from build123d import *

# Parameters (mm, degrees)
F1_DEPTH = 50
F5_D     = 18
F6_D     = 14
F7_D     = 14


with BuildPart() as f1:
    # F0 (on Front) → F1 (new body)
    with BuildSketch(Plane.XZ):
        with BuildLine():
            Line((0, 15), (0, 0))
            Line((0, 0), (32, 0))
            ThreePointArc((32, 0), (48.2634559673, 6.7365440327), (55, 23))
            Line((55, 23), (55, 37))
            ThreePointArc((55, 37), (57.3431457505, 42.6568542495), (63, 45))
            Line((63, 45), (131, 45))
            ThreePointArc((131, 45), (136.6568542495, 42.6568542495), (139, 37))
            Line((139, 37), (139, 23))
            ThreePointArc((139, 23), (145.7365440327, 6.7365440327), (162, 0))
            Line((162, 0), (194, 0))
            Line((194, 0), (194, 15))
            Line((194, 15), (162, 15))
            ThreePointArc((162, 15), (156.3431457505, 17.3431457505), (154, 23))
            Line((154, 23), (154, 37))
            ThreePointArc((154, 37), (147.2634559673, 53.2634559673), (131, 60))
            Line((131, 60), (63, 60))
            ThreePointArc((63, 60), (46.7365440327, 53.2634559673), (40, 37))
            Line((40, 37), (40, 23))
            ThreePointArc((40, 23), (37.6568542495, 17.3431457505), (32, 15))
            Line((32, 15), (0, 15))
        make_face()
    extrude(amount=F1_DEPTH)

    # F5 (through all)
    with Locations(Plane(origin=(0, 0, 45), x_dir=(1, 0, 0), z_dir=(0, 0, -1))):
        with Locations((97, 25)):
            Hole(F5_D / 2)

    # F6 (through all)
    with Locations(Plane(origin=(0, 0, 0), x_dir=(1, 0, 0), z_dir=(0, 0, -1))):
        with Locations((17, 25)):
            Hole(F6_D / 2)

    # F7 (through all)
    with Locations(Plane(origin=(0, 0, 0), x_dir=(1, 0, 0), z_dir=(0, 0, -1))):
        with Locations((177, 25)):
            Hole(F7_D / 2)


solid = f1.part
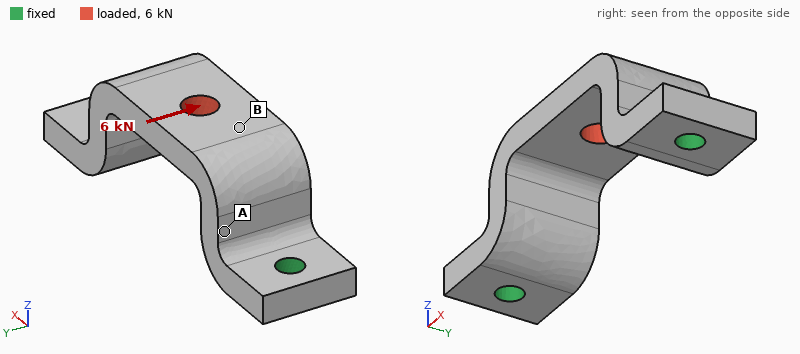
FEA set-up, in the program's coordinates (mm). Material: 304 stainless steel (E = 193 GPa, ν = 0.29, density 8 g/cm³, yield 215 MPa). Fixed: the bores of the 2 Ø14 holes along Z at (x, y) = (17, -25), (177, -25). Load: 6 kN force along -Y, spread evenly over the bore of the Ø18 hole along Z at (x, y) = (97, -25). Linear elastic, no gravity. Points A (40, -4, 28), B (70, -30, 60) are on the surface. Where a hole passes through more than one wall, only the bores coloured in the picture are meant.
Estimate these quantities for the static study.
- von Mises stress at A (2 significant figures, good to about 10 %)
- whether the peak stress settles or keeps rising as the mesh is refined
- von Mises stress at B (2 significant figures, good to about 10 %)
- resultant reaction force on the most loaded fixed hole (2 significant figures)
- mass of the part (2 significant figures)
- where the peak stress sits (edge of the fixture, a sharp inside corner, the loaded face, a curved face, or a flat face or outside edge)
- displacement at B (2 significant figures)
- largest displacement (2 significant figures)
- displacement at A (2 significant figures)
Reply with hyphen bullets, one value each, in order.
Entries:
- 19 MPa
- keeps rising
- 10 MPa
- 3.0 kN
- 1.5 kg
- edge of the fixture
- 52 µm
- 58 µm
- 27 µm
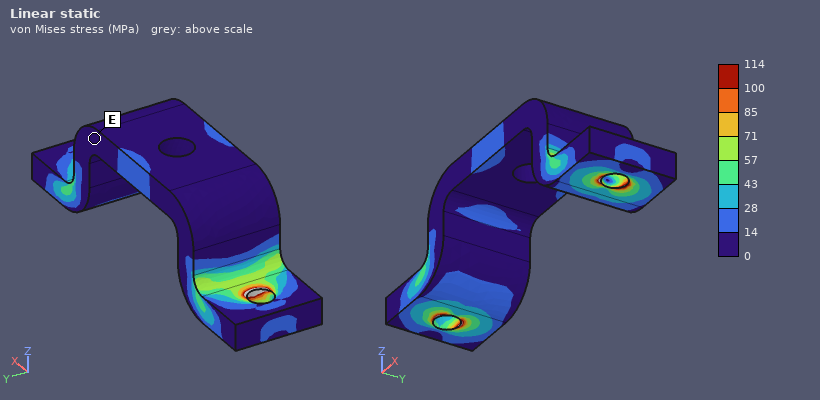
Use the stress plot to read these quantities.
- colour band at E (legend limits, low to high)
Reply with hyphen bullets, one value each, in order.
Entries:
- 0 to 14 MPa
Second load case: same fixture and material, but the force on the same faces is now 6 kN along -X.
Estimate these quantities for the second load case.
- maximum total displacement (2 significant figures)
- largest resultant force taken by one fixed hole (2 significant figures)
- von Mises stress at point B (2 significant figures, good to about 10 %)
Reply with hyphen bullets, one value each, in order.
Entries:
- 21 µm
- 3.3 kN
- 14 MPa
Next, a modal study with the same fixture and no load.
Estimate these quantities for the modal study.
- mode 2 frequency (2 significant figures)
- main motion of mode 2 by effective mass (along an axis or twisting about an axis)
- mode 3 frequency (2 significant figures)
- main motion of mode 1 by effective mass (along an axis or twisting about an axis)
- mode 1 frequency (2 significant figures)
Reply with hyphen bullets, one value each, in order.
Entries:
- 3200 Hz
- along X
- 4000 Hz
- along Y
- 2100 Hz
